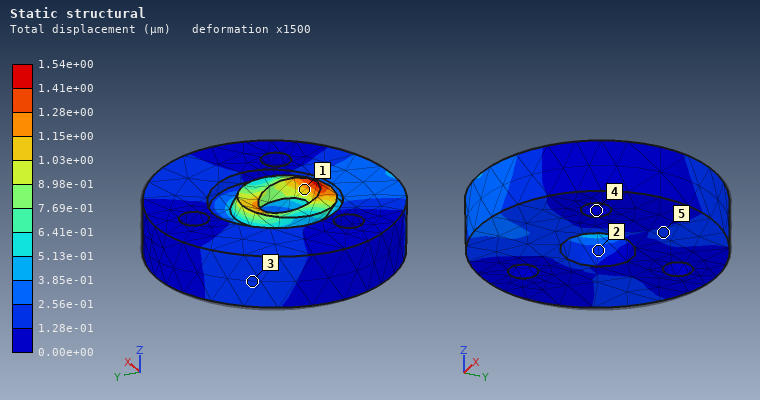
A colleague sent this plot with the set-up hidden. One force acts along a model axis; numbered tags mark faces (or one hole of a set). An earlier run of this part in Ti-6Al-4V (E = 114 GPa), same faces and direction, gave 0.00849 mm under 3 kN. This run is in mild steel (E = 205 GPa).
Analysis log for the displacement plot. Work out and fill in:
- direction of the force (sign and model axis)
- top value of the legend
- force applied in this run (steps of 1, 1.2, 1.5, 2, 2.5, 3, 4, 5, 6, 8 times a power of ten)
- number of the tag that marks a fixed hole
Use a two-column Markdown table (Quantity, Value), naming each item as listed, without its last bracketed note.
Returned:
| Quantity | Value |
|---|---|
| direction of the force | -Y |
| top value of the legend | 1.54e+00 µm |
| force applied in this run | 1 kN |
| number of the tag that marks a fixed hole | 4 |
